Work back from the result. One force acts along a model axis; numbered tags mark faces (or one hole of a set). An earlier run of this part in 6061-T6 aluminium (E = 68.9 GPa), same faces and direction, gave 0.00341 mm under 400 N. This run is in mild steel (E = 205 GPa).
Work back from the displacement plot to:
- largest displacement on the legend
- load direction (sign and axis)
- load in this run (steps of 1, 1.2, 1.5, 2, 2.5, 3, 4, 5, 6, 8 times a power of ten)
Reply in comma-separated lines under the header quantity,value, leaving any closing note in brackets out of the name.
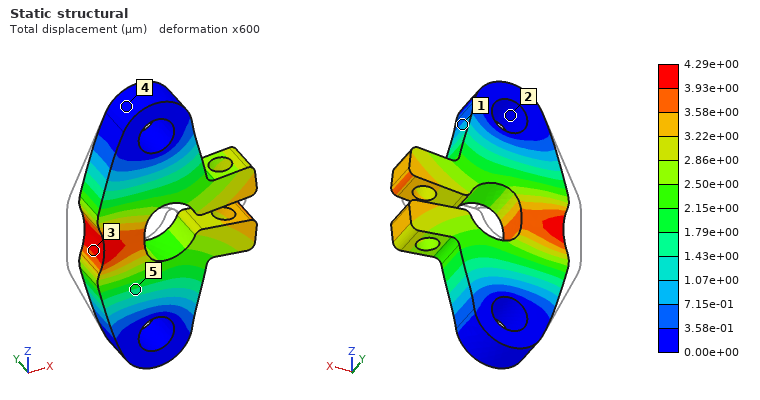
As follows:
quantity,value
largest displacement on the legend,4.29e+00 µm
load direction,+X
load in this run,1.5 kN
